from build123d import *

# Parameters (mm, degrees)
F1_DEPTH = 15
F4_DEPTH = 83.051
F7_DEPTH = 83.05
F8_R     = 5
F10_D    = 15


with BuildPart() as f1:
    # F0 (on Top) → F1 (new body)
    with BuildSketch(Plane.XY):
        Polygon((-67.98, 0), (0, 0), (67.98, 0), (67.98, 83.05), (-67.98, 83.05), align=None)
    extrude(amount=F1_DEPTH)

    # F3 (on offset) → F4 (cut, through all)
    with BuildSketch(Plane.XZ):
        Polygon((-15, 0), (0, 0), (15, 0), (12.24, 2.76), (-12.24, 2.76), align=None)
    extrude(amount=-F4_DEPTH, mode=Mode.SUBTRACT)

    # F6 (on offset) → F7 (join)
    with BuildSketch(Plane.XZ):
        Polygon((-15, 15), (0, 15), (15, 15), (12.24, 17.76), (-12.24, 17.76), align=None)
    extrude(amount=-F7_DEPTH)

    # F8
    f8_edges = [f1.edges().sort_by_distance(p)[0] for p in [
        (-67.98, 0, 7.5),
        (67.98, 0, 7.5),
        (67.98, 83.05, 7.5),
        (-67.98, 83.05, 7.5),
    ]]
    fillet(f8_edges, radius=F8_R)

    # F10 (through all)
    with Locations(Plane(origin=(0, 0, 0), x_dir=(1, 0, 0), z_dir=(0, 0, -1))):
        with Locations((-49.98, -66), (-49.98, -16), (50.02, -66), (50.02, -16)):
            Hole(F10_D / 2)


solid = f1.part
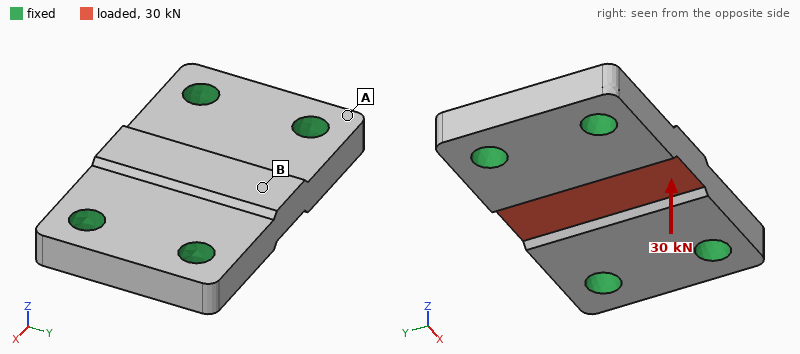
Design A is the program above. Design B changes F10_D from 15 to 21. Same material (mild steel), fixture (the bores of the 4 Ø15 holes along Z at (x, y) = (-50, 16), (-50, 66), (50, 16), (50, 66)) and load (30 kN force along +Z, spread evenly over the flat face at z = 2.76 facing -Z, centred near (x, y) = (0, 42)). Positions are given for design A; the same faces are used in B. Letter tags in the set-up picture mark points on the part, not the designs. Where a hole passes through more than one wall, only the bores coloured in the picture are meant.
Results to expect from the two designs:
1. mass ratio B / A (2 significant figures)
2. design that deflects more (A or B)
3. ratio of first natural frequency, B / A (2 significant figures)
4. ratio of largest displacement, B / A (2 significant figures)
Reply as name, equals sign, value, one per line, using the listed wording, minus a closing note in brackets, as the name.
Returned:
mass ratio B / A = 0.94
design that deflects more = A
ratio of first natural frequency, B / A = 1.2
ratio of largest displacement, B / A = 0.79
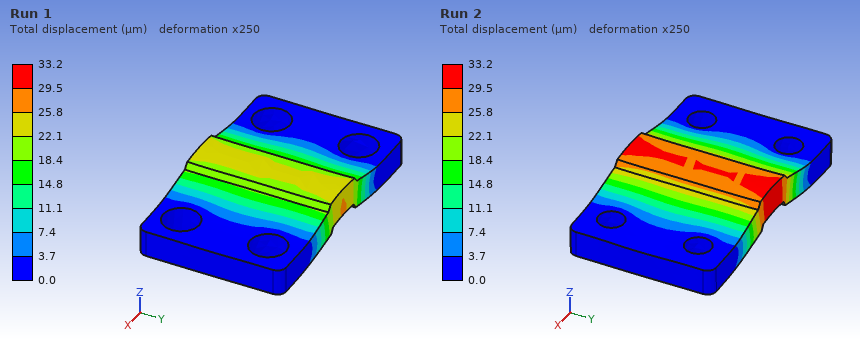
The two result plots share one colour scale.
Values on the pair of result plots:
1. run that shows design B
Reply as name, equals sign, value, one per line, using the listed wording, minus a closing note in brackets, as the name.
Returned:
run that shows design B = Run 1
